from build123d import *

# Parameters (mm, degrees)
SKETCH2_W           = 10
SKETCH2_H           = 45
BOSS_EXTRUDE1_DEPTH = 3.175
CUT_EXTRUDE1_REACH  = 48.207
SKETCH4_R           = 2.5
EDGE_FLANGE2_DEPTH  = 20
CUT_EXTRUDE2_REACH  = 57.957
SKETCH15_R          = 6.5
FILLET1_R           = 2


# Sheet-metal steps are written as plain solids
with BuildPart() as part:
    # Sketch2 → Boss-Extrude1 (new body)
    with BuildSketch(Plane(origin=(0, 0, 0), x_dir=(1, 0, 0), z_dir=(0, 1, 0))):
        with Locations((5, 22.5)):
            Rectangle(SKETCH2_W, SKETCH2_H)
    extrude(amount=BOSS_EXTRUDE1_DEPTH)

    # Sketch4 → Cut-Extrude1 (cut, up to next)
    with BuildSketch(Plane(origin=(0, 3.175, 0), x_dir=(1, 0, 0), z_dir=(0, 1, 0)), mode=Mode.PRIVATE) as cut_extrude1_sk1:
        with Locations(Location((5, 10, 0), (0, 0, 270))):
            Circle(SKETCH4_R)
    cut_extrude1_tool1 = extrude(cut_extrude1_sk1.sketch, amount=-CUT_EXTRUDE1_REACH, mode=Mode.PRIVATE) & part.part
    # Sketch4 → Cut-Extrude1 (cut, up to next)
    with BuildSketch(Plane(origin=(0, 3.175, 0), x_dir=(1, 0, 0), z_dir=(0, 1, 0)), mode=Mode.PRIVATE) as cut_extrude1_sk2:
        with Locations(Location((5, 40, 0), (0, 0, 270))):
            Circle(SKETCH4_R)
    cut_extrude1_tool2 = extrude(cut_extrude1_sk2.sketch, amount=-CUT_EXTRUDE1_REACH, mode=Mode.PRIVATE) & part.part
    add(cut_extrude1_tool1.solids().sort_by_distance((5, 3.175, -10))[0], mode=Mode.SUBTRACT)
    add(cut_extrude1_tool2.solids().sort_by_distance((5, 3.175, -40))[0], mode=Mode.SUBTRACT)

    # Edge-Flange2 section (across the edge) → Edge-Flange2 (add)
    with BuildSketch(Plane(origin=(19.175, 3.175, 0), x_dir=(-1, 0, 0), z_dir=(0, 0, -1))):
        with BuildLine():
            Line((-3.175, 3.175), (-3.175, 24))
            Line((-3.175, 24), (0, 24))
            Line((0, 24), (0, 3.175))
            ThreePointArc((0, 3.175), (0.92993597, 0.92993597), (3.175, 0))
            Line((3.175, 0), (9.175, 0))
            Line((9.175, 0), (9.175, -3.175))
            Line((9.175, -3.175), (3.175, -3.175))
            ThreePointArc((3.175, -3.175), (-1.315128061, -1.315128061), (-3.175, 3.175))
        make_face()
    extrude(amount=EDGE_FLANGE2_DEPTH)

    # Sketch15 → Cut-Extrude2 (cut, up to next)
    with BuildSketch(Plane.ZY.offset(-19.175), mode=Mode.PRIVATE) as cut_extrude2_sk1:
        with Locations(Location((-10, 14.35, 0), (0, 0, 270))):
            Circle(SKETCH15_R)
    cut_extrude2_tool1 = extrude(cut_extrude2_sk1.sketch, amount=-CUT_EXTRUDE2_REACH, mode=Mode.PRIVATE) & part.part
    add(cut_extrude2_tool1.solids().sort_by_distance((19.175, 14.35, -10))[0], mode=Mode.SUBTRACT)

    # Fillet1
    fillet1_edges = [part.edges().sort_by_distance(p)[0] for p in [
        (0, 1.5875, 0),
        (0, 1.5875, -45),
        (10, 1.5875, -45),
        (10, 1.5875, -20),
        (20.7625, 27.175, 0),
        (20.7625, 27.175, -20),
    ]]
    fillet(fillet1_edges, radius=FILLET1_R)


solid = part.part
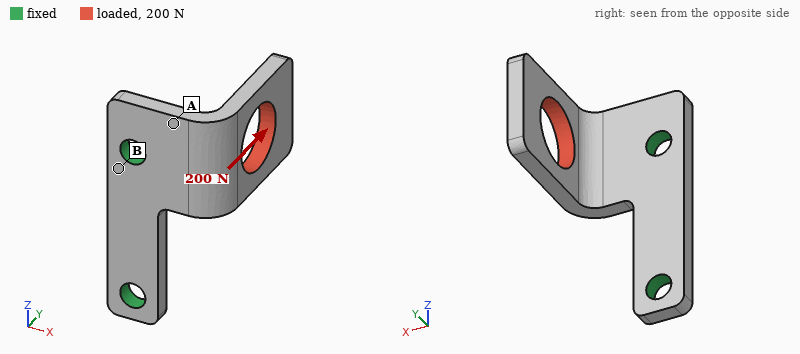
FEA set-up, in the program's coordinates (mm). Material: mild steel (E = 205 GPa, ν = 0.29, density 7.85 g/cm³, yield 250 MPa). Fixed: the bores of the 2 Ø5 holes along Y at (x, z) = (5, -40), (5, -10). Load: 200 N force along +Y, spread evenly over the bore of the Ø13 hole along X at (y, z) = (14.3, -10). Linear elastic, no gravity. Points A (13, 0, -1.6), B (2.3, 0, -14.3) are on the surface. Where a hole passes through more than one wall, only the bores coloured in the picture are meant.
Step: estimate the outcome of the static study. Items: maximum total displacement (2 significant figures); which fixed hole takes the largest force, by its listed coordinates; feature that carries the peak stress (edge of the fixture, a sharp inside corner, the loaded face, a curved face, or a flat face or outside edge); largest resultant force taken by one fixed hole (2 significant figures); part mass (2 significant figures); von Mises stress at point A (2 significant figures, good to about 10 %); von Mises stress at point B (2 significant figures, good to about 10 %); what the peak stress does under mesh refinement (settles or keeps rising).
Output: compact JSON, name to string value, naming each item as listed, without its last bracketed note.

{"maximum total displacement": "56 µm", "which fixed hole takes the largest force, by its listed coordinates": "(5, -10)", "feature that carries the peak stress": "edge of the fixture", "largest resultant force taken by one fixed hole": "200 N", "part mass": "24 g", "von Mises stress at point A": "40 MPa", "von Mises stress at point B": "14 MPa", "what the peak stress does under mesh refinement": "keeps rising"}
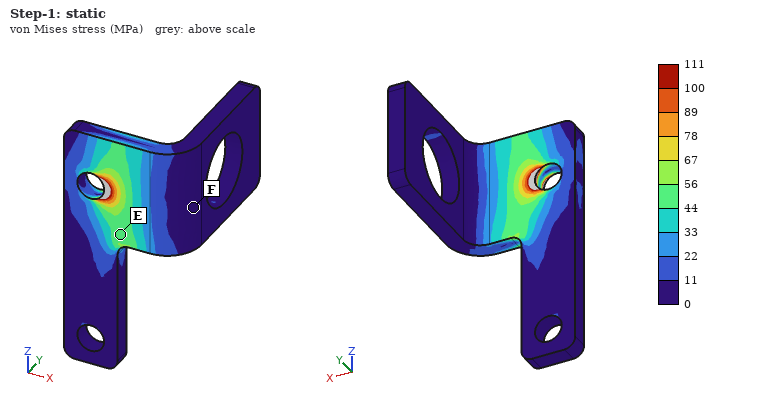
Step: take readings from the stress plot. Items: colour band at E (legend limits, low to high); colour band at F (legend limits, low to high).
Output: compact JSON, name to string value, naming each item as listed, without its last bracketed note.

{"colour band at E": "44 to 56 MPa", "colour band at F": "0 to 11 MPa"}
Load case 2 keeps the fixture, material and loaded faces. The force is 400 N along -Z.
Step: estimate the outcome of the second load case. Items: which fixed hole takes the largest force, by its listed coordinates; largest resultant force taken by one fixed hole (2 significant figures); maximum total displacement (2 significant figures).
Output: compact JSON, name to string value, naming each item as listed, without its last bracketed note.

{"which fixed hole takes the largest force, by its listed coordinates": "(5, -10)", "largest resultant force taken by one fixed hole": "340 N", "maximum total displacement": "0.11 mm"}
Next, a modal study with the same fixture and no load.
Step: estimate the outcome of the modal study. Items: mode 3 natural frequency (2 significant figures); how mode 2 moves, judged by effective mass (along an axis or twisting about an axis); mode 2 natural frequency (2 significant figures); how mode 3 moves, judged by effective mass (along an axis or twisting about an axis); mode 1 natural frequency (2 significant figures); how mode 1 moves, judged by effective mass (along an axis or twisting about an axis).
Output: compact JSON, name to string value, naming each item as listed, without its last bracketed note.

{"mode 3 natural frequency": "6700 Hz", "how mode 2 moves, judged by effective mass": "along Z", "mode 2 natural frequency": "3500 Hz", "how mode 3 moves, judged by effective mass": "along Y", "mode 1 natural frequency": "2300 Hz", "how mode 1 moves, judged by effective mass": "along X"}
